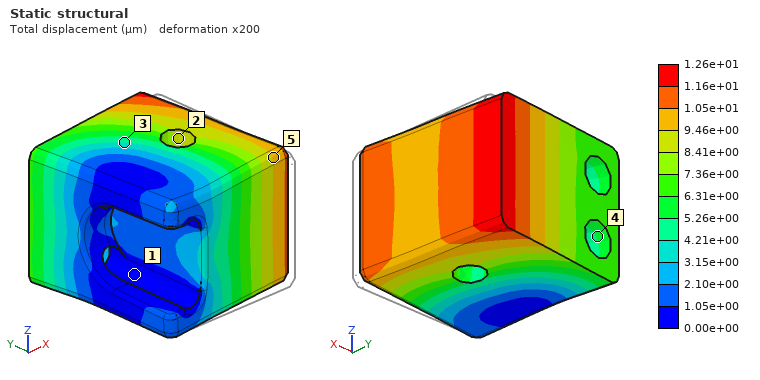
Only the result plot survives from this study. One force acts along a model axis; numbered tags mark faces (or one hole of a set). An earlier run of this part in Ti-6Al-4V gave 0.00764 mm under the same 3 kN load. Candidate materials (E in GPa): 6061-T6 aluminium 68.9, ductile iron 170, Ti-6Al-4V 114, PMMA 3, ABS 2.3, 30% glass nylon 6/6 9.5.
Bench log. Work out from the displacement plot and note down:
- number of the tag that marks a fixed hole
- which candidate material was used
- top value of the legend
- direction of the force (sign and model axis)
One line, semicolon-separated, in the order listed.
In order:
1; 6061-T6 aluminium; 1.26e+01 µm; +Y
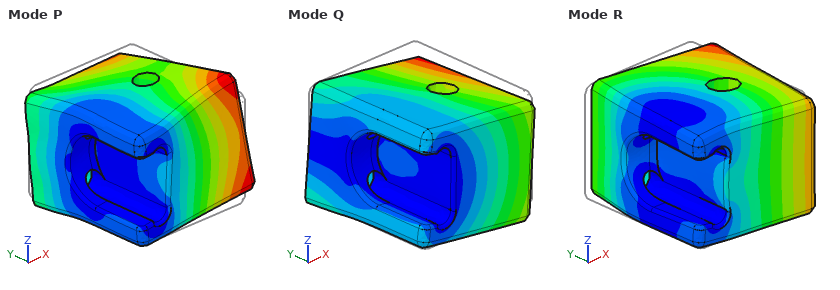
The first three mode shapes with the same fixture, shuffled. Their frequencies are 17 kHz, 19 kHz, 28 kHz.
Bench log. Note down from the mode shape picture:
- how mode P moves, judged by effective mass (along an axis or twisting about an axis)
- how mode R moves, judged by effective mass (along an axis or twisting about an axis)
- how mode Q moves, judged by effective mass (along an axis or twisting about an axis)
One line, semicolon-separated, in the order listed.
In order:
twisting about X; along Y; along Z
